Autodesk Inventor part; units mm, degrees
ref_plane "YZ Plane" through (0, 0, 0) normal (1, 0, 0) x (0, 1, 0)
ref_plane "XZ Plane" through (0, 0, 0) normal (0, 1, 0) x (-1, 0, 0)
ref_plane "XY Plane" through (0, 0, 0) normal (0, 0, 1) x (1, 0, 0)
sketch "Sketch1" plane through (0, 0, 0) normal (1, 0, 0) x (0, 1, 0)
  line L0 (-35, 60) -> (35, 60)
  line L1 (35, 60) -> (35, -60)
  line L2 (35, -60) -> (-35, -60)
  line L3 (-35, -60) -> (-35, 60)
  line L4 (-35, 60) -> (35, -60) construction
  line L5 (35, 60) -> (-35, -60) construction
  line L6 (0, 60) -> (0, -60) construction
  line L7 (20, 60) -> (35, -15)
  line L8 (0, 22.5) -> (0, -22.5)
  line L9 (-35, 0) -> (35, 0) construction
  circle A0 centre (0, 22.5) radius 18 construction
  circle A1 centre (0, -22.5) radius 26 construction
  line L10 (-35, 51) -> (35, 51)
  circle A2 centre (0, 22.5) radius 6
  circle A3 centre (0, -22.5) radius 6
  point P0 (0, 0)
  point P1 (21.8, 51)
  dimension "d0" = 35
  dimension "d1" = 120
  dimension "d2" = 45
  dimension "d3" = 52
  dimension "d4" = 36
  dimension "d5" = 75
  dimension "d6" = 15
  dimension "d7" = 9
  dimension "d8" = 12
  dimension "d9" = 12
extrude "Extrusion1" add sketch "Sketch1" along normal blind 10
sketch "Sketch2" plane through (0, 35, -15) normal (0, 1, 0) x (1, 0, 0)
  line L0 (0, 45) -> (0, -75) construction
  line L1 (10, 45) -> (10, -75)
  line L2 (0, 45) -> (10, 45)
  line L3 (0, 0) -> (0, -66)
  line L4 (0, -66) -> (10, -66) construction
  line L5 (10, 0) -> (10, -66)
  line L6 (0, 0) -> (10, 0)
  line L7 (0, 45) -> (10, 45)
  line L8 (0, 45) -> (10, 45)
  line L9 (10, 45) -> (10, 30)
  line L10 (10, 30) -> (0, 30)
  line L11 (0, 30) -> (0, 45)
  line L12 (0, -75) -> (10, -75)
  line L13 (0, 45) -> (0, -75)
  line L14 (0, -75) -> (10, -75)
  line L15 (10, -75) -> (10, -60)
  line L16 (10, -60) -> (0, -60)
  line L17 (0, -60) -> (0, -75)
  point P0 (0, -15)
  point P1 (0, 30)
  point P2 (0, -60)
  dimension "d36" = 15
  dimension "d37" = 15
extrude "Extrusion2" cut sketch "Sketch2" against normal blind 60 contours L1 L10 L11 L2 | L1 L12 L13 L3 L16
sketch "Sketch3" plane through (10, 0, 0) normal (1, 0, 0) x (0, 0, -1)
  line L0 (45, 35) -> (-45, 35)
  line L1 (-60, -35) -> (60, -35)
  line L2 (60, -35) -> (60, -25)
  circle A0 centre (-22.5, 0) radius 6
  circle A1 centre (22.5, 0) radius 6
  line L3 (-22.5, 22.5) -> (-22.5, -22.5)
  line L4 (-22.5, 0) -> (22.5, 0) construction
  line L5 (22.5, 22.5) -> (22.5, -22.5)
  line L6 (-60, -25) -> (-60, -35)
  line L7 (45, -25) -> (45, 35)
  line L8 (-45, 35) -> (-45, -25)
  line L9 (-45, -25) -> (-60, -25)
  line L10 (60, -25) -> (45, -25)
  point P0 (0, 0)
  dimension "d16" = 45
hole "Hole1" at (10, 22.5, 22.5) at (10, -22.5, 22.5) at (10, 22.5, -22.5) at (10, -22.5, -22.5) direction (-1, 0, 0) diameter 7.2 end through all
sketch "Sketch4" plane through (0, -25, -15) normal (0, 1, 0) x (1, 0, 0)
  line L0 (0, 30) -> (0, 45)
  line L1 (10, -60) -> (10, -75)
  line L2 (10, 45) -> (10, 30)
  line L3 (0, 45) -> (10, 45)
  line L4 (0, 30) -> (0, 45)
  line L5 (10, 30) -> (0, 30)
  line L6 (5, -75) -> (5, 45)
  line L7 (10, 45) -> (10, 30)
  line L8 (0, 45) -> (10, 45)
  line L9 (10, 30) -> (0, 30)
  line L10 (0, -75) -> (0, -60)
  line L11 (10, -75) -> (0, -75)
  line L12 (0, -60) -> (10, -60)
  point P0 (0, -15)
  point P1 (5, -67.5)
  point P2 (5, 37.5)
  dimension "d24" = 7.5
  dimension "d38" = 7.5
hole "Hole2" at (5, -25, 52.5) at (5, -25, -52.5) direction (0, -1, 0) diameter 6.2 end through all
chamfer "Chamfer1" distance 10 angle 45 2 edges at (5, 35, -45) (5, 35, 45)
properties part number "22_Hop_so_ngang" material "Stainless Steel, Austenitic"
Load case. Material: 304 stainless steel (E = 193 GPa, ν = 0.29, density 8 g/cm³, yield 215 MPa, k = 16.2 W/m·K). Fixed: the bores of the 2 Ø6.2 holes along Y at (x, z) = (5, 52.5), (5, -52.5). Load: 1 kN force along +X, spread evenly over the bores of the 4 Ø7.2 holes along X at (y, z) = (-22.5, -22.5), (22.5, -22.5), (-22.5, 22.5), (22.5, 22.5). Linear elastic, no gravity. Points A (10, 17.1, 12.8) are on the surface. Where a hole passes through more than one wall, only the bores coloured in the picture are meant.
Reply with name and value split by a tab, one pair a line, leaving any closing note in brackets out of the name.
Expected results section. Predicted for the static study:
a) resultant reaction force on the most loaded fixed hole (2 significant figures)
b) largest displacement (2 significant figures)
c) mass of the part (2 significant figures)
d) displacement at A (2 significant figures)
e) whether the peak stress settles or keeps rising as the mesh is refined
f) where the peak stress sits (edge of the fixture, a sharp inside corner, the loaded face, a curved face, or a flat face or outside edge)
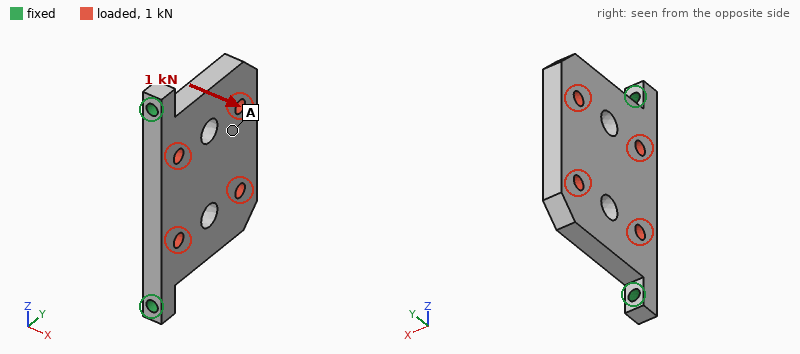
resultant reaction force on the most loaded fixed hole	500 N
largest displacement	0.13 mm
mass of the part	480 g
displacement at A	0.092 mm
whether the peak stress settles or keeps rising as the mesh is refined	keeps rising
where the peak stress sits	edge of the fixture
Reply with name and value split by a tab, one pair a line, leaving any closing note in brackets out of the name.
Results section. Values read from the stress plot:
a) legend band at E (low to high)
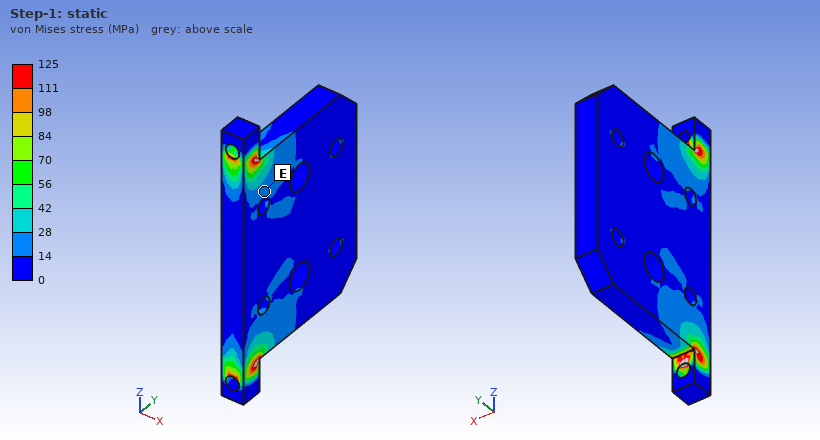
legend band at E	14 to 28 MPa
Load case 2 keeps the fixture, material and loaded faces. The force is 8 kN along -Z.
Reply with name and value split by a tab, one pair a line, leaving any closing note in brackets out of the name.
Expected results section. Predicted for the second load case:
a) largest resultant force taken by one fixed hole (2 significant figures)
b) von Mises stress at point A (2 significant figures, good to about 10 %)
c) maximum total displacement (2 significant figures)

largest resultant force taken by one fixed hole	4.7 kN
von Mises stress at point A	8.5 MPa
maximum total displacement	15 µm
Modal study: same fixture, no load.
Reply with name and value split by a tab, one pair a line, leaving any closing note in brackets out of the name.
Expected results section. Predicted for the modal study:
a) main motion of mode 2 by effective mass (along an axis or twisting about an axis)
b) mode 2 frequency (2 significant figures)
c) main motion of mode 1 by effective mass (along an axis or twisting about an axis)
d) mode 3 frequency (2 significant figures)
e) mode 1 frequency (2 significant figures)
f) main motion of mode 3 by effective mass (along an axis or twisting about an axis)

main motion of mode 2 by effective mass	twisting about Y
mode 2 frequency	2900 Hz
main motion of mode 1 by effective mass	along X
mode 3 frequency	4000 Hz
mode 1 frequency	820 Hz
main motion of mode 3 by effective mass	along X
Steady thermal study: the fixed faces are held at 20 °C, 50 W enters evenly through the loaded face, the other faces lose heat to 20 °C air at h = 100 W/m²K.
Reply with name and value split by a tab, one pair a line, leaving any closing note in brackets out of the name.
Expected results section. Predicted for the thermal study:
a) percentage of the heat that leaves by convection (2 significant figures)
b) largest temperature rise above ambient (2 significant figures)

percentage of the heat that leaves by convection	89 %
largest temperature rise above ambient	50 K
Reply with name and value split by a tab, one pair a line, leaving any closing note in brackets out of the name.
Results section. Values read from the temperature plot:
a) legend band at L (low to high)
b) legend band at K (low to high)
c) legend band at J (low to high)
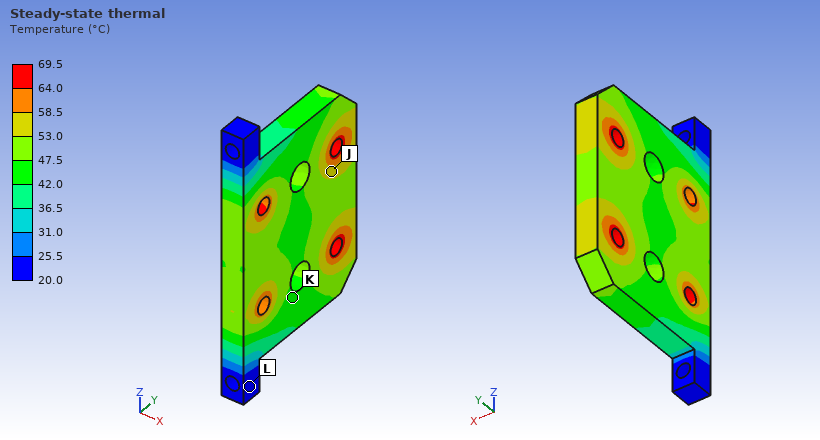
legend band at L	20.0 to 25.5 °C
legend band at K	42.0 to 47.5 °C
legend band at J	53.0 to 58.5 °C
